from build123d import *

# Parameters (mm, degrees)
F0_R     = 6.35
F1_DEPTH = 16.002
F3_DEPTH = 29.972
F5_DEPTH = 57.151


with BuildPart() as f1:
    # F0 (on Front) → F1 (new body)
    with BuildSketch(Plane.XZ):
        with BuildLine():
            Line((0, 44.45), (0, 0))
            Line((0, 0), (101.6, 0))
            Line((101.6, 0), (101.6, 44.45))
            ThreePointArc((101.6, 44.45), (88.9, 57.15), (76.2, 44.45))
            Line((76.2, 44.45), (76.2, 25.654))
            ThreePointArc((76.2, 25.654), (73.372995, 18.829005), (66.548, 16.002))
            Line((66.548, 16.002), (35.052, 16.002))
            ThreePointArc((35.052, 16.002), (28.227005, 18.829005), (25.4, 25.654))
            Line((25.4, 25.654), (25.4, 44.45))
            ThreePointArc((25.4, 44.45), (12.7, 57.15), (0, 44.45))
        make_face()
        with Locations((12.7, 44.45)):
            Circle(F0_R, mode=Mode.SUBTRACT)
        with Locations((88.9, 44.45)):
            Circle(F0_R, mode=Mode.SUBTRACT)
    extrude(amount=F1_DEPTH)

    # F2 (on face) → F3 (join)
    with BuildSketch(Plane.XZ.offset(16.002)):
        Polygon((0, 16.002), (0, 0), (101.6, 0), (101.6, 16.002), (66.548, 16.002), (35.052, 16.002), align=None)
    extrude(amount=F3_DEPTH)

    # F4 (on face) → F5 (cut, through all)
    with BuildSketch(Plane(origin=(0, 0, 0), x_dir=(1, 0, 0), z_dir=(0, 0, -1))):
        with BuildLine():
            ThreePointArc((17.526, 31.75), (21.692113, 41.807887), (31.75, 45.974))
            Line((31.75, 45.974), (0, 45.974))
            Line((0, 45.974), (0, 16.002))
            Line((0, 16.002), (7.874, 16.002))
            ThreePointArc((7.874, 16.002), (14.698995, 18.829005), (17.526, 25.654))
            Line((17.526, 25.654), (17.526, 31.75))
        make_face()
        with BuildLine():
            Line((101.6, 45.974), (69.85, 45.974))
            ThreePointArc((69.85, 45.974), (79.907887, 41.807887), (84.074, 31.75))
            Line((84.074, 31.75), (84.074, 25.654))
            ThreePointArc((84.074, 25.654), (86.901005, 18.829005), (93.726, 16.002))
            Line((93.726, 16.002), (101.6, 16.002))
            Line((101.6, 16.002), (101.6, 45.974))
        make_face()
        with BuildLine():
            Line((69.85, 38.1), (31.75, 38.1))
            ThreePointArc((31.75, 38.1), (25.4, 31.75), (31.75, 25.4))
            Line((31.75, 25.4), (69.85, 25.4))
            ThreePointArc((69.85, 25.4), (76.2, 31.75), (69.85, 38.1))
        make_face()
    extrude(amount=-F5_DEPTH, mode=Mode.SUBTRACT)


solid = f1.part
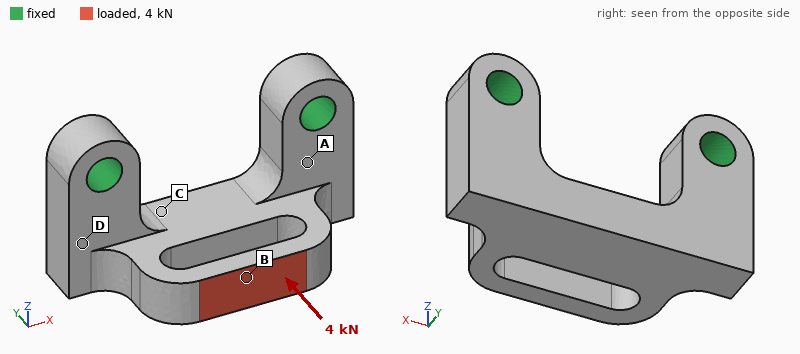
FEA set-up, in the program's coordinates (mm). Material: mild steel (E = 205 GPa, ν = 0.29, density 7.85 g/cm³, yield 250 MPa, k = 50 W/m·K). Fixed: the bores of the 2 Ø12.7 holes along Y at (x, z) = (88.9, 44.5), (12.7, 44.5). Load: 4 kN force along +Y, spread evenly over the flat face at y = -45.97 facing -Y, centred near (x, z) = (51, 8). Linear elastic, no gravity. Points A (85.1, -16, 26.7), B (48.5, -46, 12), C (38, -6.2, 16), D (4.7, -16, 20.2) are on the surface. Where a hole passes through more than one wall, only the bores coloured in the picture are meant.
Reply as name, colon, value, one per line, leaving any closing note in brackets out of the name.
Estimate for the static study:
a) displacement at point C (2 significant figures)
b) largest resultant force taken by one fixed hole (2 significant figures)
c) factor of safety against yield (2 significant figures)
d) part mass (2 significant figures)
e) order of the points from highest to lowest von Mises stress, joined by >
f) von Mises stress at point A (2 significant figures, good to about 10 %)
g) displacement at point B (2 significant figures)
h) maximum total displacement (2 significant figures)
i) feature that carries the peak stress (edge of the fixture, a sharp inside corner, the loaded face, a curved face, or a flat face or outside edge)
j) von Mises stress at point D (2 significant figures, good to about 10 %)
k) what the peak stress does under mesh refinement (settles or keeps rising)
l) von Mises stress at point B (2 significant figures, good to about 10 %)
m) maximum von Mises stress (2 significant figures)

displacement at point C: 10 µm
largest resultant force taken by one fixed hole: 2.0 kN
factor of safety against yield: 1.8
part mass: 590 g
order of the points from highest to lowest von Mises stress, joined by >: B > A > D > C
von Mises stress at point A: 35 MPa
displacement at point B: 47 µm
maximum total displacement: 56 µm
feature that carries the peak stress: a curved face
von Mises stress at point D: 21 MPa
what the peak stress does under mesh refinement: settles
von Mises stress at point B: 97 MPa
maximum von Mises stress: 140 MPa
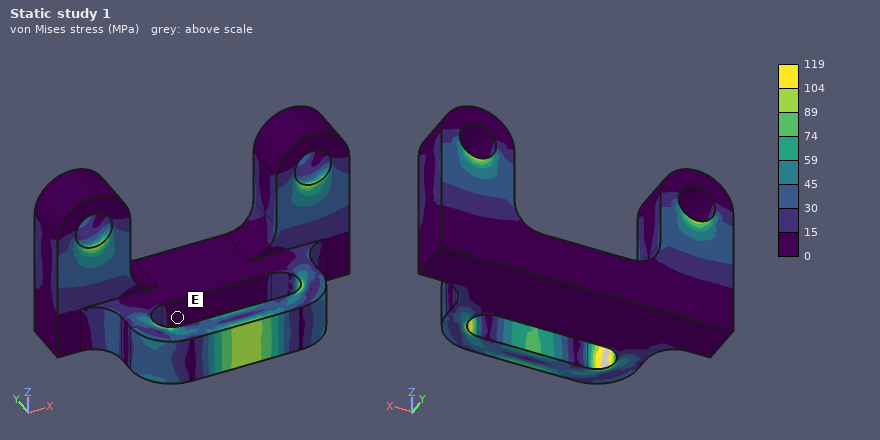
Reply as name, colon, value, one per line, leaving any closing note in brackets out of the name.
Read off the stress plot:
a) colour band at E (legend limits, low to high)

colour band at E: 0 to 15 MPa
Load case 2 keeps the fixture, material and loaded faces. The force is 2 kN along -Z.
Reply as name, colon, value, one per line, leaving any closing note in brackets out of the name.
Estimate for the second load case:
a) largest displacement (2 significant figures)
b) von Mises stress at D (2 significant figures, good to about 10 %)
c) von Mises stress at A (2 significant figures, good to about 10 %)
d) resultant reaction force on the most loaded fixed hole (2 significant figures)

largest displacement: 61 µm
von Mises stress at D: 27 MPa
von Mises stress at A: 39 MPa
resultant reaction force on the most loaded fixed hole: 1.1 kN
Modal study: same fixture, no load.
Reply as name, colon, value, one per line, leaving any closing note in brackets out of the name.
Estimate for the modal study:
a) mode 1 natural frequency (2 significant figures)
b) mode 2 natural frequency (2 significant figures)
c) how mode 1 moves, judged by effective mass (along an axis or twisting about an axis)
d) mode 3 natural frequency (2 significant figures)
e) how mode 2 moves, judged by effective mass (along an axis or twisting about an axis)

mode 1 natural frequency: 3200 Hz
mode 2 natural frequency: 5600 Hz
how mode 1 moves, judged by effective mass: along Y
mode 3 natural frequency: 6800 Hz
how mode 2 moves, judged by effective mass: along X
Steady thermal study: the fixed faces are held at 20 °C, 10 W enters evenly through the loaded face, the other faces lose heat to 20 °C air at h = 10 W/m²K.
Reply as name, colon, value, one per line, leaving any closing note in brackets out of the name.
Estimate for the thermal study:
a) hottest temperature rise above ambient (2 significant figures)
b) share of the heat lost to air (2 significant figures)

hottest temperature rise above ambient: 35 K
share of the heat lost to air: 14 %
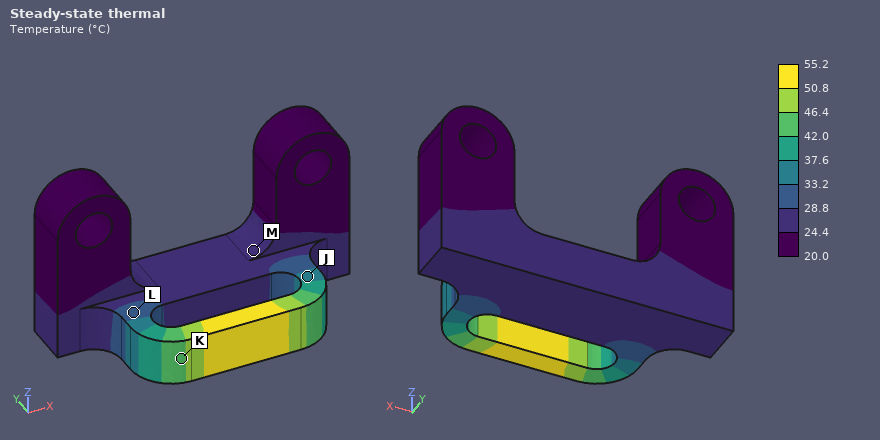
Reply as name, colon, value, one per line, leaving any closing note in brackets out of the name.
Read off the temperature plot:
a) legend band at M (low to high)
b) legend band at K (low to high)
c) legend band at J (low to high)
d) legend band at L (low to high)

legend band at M: 24.4 to 28.8 °C
legend band at K: 42.0 to 46.4 °C
legend band at J: 33.2 to 37.6 °C
legend band at L: 28.8 to 33.2 °C
